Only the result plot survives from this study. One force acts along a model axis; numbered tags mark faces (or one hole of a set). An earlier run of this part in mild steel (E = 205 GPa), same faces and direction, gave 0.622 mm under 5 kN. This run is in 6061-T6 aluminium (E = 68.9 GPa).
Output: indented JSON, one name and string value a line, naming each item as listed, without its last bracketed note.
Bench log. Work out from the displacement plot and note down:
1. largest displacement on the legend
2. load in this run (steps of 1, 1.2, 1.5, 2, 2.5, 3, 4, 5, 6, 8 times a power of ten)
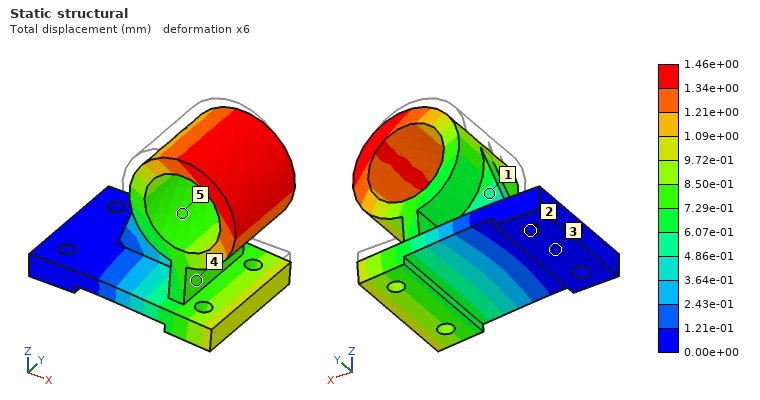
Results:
{
  "largest displacement on the legend": "1.46e+00 mm",
  "load in this run": "4 kN"
}
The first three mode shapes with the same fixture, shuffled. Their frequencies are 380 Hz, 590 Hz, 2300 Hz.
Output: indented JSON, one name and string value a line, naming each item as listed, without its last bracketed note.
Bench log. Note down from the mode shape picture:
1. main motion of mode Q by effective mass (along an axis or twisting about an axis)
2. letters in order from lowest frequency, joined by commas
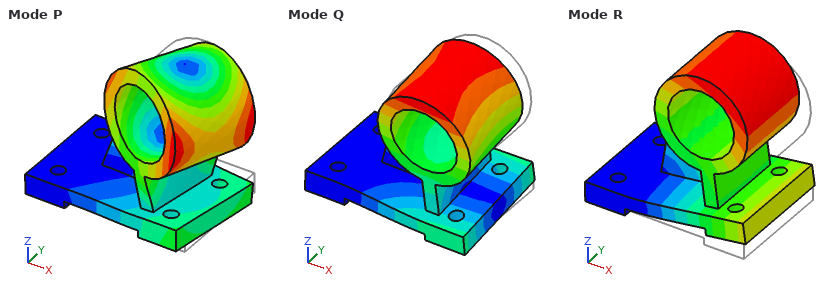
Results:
{
  "main motion of mode Q by effective mass": "along Y",
  "letters in order from lowest frequency, joined by commas": "R, Q, P"
}
